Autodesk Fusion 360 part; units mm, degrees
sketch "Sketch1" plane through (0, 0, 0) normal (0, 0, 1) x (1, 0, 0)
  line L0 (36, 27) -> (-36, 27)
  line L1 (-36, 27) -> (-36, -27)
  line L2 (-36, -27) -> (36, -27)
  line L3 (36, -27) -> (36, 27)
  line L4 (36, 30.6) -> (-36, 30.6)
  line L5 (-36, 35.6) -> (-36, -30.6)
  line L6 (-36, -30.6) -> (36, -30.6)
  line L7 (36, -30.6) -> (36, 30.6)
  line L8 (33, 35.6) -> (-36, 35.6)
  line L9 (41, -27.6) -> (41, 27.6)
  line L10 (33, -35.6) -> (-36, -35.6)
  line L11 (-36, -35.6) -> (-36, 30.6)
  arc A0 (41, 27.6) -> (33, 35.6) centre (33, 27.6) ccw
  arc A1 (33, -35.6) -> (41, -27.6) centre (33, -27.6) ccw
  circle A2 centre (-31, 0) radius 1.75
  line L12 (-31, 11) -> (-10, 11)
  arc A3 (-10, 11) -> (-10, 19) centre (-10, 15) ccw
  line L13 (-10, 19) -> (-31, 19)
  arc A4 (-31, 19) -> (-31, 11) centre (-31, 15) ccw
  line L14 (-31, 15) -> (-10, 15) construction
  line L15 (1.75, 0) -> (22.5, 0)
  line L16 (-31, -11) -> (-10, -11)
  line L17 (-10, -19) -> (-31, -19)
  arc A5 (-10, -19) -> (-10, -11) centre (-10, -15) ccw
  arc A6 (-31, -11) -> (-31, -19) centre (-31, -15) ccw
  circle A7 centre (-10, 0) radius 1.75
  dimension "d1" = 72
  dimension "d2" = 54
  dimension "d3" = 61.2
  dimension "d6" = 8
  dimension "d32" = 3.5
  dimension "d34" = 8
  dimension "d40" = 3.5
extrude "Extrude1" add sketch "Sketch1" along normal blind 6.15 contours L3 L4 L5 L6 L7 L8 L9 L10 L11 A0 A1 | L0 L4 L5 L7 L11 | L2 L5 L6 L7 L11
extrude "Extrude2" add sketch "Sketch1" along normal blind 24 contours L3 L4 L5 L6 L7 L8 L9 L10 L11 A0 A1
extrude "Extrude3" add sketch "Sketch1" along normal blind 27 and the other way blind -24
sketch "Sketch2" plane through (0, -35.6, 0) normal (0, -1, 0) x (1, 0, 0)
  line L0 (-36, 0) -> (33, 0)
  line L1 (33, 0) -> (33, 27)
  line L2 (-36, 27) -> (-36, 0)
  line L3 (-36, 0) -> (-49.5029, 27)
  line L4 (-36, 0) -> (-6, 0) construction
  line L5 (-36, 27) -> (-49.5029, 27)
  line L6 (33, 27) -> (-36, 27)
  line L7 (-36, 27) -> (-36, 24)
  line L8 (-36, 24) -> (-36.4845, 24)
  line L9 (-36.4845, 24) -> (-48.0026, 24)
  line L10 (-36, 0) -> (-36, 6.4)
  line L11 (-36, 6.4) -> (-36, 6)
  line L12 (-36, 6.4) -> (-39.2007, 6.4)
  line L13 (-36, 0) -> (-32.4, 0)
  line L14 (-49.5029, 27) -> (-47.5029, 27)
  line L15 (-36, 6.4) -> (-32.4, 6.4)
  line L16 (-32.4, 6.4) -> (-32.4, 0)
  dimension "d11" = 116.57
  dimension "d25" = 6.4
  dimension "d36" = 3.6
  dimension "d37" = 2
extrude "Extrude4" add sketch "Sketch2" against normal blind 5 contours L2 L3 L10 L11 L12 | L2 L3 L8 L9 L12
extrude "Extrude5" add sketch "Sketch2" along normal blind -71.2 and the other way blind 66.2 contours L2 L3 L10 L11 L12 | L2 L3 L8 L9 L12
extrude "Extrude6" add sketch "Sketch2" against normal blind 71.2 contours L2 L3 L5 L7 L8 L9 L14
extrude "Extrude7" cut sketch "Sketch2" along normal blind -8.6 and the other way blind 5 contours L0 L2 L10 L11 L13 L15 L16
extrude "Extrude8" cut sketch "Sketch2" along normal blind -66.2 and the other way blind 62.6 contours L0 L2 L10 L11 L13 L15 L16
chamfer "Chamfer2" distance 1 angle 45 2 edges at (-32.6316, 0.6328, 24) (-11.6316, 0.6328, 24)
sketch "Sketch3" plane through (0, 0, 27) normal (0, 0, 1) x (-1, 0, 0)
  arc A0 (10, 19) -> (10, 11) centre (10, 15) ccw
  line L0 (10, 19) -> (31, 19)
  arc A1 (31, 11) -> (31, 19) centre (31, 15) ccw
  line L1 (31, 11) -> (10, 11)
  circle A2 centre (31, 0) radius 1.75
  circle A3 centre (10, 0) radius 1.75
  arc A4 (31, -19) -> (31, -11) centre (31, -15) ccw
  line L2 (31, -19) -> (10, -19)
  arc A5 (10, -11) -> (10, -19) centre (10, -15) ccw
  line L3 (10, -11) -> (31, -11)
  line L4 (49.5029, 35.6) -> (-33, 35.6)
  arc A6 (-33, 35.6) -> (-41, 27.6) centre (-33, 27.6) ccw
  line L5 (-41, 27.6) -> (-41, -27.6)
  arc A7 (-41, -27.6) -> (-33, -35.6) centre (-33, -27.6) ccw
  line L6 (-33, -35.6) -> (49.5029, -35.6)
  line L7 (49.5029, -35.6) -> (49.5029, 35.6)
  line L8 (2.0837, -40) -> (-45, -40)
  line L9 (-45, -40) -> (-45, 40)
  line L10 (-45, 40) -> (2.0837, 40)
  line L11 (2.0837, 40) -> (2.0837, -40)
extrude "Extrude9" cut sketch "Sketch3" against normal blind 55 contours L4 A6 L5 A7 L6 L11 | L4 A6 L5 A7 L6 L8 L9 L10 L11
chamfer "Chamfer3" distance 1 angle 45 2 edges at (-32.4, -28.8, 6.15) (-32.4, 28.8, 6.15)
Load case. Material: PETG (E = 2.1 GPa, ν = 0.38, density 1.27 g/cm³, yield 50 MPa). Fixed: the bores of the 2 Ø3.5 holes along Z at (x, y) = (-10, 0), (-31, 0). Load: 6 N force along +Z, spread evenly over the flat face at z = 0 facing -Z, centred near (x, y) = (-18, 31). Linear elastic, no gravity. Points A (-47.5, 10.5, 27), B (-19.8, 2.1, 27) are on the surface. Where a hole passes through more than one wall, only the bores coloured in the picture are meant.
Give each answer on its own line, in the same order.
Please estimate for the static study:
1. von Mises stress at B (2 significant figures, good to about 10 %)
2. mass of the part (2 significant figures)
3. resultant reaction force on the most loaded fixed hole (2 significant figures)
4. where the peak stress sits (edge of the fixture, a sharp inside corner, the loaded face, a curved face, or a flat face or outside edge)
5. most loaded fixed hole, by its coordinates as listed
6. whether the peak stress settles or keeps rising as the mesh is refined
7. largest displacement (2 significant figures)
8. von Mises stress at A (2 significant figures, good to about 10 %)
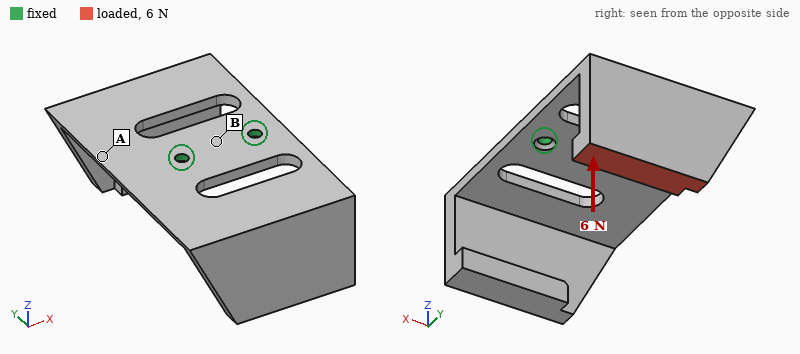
0.84 MPa
25 g
3.6 N
edge of the fixture
(-10, 0)
keeps rising
1.0 mm
2.6 MPa
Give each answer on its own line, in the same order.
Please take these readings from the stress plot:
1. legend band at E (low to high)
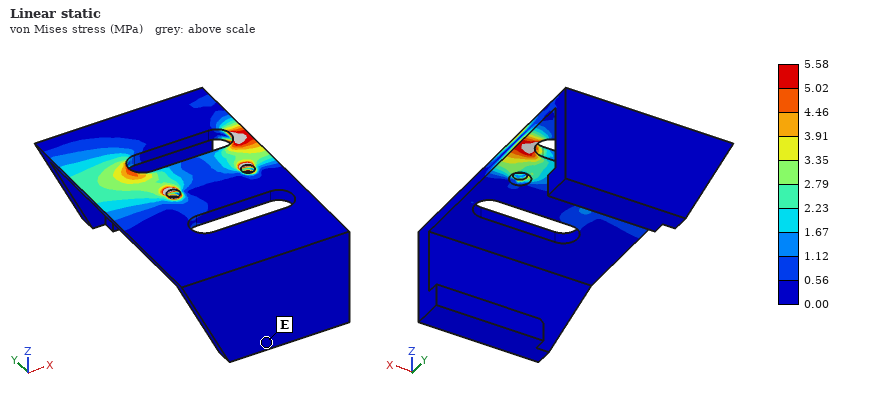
0.00 to 0.56 MPa
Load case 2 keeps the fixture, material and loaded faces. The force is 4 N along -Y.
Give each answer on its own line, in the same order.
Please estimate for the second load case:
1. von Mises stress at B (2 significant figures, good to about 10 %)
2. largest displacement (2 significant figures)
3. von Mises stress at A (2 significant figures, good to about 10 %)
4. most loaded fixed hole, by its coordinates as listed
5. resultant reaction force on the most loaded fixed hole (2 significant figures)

0.47 MPa
0.96 mm
2.5 MPa
(-10, 0)
2.5 N
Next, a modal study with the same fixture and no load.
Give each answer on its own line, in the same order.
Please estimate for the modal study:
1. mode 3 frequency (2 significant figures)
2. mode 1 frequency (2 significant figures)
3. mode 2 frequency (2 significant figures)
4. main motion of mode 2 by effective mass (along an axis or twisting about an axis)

320 Hz
130 Hz
140 Hz
along Z
